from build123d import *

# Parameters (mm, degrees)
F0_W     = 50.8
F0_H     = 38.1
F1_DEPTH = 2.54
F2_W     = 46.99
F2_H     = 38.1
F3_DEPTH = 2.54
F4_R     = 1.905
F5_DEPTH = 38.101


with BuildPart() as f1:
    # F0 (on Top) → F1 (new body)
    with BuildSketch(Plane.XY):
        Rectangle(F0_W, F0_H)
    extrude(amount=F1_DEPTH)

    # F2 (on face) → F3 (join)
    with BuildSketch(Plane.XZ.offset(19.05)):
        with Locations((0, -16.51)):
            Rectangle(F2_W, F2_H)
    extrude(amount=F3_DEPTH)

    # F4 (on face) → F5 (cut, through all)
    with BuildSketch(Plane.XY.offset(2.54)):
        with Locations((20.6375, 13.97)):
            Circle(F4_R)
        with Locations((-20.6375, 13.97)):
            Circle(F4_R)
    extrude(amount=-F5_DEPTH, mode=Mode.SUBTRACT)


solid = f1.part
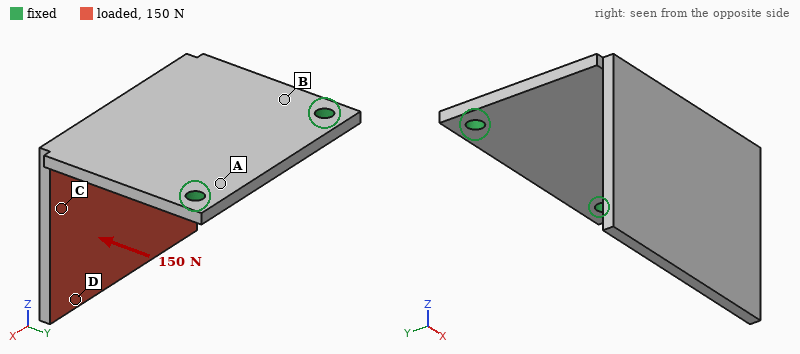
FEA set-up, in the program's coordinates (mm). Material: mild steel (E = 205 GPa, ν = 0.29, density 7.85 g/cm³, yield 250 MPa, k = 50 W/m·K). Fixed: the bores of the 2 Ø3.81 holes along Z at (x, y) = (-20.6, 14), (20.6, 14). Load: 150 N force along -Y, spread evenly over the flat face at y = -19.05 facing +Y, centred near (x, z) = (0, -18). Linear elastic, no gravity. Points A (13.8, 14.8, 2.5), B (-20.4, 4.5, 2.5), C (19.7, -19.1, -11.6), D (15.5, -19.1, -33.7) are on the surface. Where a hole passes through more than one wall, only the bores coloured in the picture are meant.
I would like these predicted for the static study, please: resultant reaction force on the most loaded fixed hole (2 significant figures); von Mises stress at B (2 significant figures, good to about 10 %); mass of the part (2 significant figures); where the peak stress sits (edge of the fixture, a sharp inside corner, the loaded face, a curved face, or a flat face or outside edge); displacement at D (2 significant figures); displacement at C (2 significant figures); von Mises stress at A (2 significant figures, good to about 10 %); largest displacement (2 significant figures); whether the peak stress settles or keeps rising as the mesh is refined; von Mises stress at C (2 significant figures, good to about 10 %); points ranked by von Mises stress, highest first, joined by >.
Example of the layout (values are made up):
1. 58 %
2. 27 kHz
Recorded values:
1. 79 N
2. 57 MPa
3. 74 g
4. edge of the fixture
5. 0.33 mm
6. 0.16 mm
7. 41 MPa
8. 0.36 mm
9. keeps rising
10. 22 MPa
11. B > A > C > D
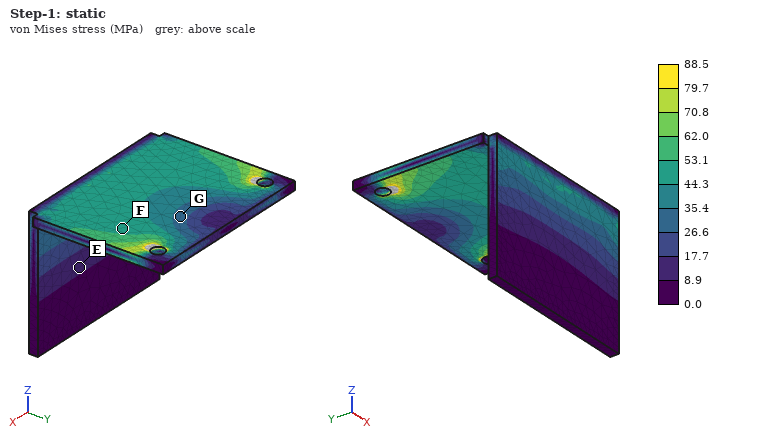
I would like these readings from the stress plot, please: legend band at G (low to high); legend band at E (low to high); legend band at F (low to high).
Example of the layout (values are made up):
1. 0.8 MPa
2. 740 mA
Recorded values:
1. 26.6 to 35.4 MPa
2. 8.9 to 17.7 MPa
3. 44.3 to 53.1 MPa
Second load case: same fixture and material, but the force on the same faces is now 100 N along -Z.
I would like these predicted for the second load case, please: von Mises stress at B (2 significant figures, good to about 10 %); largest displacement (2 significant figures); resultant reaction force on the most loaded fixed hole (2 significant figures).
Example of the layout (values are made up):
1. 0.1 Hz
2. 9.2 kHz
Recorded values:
1. 50 MPa
2. 0.20 mm
3. 50 N
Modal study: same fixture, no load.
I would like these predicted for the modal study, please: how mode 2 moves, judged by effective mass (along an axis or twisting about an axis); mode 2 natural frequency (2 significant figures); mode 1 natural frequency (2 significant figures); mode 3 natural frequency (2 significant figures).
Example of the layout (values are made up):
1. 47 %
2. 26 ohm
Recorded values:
1. along X
2. 1100 Hz
3. 540 Hz
4. 1500 Hz
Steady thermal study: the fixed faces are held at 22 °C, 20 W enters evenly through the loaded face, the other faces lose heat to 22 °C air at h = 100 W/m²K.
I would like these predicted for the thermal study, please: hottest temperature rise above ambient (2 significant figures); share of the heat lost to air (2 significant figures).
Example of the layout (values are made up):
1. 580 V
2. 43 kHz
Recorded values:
1. 60 K
2. 83 %
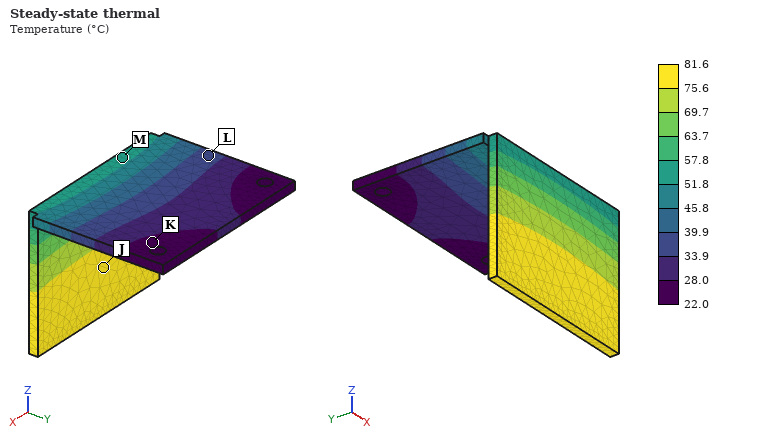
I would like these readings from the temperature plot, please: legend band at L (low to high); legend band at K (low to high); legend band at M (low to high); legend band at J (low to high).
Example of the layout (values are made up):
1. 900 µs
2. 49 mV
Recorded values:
1. 33.9 to 39.9 °C
2. 22.0 to 28.0 °C
3. 51.8 to 57.8 °C
4. 75.6 to 81.6 °C
